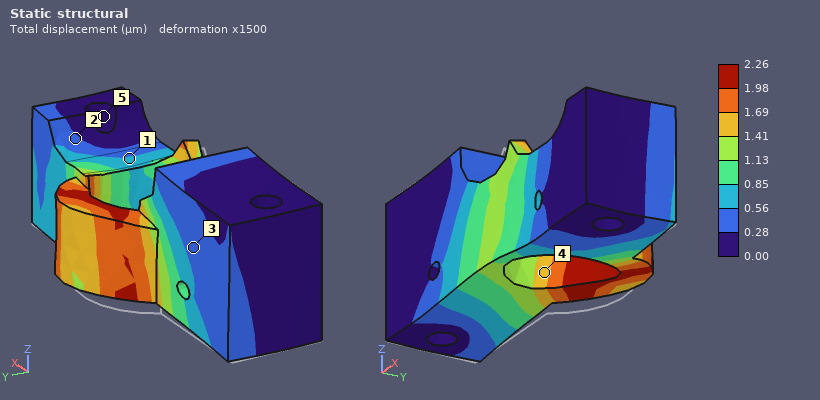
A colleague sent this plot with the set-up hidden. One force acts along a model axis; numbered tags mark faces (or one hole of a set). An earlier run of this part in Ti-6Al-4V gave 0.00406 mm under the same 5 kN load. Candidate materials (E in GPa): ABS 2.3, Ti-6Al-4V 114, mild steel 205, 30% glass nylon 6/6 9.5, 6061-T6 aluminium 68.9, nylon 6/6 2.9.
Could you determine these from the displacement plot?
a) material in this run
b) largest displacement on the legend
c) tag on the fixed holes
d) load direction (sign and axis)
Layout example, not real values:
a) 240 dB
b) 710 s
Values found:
a) mild steel
b) 2.26 µm
c) 5
d) +X
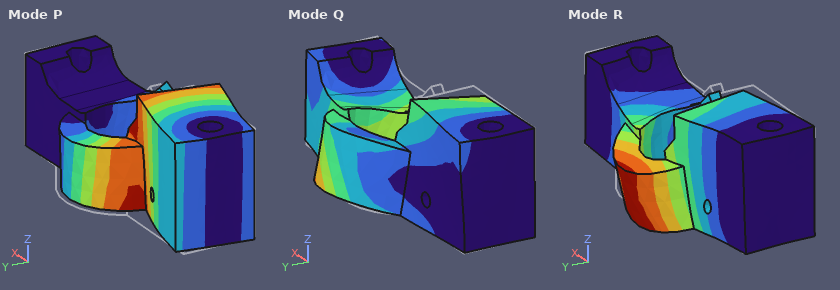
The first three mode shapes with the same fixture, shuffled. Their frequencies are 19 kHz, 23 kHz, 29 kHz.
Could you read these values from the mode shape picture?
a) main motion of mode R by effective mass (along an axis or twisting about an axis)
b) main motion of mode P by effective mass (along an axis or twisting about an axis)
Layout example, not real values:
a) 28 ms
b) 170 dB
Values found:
a) along Z
b) along Y
